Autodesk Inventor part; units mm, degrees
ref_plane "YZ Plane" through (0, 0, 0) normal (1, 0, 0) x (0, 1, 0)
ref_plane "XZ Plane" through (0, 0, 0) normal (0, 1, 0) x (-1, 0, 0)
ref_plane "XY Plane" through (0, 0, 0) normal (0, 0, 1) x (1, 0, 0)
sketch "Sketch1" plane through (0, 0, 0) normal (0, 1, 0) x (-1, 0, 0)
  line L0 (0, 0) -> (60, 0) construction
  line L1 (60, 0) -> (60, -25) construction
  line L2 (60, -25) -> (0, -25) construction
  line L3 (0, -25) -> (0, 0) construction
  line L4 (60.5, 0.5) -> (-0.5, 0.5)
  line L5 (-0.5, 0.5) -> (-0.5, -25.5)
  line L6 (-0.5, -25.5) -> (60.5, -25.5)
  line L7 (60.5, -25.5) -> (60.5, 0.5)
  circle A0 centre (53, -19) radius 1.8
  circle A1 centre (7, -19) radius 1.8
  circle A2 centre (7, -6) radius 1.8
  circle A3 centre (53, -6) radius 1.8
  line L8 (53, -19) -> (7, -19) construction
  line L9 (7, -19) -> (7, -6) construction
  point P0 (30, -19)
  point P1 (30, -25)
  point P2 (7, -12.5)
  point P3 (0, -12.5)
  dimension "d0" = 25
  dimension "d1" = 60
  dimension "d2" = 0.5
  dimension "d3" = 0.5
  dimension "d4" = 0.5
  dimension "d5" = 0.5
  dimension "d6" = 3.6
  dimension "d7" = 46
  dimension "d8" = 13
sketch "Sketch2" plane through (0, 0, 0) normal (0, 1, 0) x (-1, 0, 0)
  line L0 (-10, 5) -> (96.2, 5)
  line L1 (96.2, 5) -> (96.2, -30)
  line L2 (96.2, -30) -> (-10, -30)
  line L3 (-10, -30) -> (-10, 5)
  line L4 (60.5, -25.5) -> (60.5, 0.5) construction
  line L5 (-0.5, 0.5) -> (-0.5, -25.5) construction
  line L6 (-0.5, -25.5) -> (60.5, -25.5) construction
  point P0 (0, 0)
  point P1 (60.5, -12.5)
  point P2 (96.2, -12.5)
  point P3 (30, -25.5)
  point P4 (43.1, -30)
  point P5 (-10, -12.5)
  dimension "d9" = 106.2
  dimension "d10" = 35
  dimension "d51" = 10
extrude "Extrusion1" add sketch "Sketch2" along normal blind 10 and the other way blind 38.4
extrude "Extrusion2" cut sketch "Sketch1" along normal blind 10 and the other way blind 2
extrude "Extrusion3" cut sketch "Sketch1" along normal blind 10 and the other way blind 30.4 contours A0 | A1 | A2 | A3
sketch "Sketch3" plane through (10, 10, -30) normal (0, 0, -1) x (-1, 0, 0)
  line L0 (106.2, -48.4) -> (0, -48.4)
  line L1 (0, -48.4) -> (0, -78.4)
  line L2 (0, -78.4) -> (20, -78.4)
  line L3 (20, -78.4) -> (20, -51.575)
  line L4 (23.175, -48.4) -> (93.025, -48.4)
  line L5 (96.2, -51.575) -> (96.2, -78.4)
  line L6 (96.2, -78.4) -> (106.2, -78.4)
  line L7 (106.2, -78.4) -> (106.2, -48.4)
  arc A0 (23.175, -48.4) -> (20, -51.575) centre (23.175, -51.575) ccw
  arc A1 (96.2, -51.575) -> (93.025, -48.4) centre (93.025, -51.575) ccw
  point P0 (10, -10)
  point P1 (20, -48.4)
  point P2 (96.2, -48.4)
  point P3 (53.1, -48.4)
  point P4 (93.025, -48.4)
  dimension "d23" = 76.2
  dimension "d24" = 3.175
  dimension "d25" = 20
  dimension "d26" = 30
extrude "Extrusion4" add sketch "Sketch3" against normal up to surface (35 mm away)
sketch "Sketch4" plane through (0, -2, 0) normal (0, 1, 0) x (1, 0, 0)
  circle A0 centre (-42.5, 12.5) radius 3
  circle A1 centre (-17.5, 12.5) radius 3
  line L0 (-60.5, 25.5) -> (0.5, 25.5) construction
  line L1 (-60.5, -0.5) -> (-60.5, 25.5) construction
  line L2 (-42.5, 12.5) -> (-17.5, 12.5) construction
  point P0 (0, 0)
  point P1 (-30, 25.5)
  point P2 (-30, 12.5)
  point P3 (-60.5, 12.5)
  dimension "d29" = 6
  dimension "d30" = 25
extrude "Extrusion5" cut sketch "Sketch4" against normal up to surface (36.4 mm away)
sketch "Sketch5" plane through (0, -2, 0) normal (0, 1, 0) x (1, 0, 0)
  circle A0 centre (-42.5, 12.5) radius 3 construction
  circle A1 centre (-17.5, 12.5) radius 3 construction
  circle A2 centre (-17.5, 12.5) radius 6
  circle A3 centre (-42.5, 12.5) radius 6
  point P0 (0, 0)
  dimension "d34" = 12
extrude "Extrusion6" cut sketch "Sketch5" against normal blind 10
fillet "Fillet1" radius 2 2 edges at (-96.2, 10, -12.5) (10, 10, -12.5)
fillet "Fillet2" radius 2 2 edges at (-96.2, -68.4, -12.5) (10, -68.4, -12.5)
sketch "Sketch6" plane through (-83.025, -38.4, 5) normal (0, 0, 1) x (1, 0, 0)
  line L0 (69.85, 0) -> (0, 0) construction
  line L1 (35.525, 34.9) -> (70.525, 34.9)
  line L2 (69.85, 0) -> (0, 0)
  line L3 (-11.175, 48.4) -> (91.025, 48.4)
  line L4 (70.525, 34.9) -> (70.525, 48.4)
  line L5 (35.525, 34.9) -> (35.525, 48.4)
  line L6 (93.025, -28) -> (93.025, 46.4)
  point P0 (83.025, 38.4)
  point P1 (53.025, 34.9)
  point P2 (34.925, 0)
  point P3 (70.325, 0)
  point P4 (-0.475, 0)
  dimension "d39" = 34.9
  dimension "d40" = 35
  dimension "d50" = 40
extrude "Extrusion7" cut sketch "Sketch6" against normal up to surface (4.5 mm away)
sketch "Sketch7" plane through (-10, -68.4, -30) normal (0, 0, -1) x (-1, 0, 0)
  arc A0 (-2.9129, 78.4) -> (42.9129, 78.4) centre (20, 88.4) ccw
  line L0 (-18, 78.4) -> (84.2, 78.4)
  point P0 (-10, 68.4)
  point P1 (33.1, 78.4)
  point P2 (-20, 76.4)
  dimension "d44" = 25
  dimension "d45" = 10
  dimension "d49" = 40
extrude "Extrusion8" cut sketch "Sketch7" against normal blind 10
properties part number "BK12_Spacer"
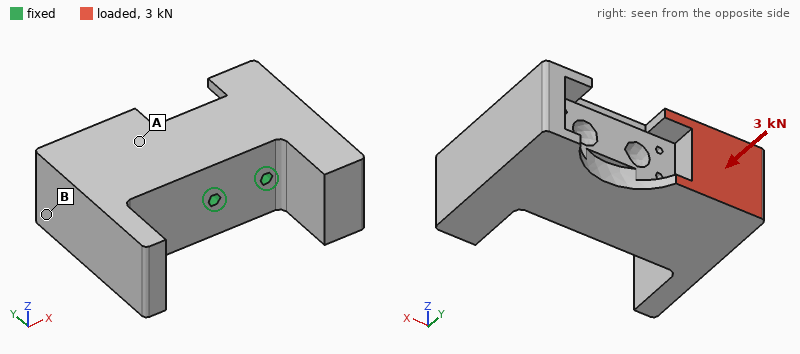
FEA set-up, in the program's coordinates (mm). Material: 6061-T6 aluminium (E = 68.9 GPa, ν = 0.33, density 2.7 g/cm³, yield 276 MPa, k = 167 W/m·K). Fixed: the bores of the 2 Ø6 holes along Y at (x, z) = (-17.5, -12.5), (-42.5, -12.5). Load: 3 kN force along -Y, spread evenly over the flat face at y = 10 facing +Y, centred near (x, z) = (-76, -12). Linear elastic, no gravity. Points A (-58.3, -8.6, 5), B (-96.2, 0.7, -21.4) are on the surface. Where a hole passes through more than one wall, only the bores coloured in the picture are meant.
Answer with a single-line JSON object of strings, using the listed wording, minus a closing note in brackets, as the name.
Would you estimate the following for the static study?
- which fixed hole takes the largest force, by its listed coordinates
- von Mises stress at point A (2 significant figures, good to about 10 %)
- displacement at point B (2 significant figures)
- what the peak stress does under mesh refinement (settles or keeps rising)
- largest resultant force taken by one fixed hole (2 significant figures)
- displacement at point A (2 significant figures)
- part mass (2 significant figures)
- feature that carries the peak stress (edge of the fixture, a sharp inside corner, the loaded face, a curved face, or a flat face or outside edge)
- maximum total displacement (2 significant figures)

{"which fixed hole takes the largest force, by its listed coordinates": "(-42.5, -12.5)", "von Mises stress at point A": "6.6 MPa", "displacement at point B": "22 µm", "what the peak stress does under mesh refinement": "keeps rising", "largest resultant force taken by one fixed hole": "4.2 kN", "displacement at point A": "7.3 µm", "part mass": "490 g", "feature that carries the peak stress": "edge of the fixture", "maximum total displacement": "25 µm"}
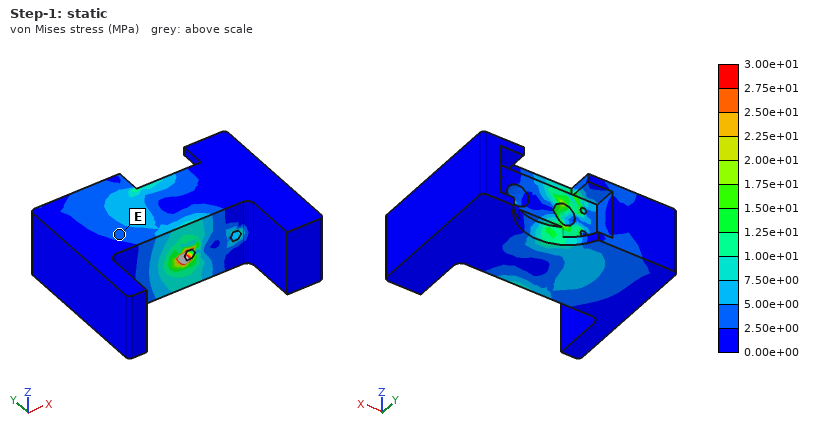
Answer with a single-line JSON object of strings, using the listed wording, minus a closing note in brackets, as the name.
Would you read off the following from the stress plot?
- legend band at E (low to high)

{"legend band at E": "2.50e+00 to 5.00e+00 MPa"}
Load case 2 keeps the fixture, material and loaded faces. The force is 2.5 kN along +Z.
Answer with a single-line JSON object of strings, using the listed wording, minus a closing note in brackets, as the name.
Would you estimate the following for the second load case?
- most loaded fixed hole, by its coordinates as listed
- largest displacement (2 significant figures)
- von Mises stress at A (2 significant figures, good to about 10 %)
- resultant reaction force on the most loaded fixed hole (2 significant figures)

{"most loaded fixed hole, by its coordinates as listed": "(-42.5, -12.5)", "largest displacement": "39 µm", "von Mises stress at A": "12 MPa", "resultant reaction force on the most loaded fixed hole": "5.0 kN"}
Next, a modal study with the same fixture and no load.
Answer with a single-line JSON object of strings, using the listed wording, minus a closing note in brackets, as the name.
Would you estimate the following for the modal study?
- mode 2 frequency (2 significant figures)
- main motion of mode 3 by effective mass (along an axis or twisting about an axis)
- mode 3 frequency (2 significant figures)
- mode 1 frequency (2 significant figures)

{"mode 2 frequency": "4100 Hz", "main motion of mode 3 by effective mass": "twisting about X", "mode 3 frequency": "5700 Hz", "mode 1 frequency": "4000 Hz"}
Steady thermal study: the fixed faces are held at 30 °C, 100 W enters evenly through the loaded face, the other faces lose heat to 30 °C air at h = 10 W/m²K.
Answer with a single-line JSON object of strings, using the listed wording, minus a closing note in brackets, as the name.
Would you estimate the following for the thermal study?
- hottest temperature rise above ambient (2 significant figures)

{"hottest temperature rise above ambient": "26 K"}
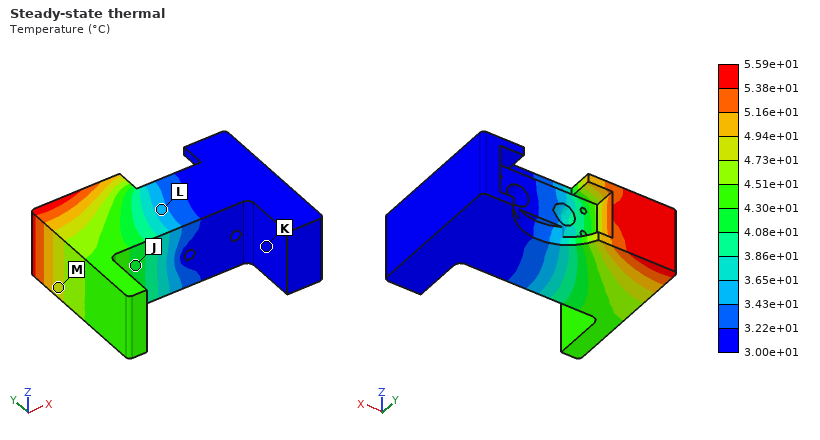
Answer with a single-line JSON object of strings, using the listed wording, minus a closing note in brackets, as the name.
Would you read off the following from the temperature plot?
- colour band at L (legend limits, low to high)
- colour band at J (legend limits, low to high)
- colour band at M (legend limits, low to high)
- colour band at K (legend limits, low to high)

{"colour band at L": "3.43e+01 to 3.65e+01 °C", "colour band at J": "4.08e+01 to 4.30e+01 °C", "colour band at M": "4.73e+01 to 4.94e+01 °C", "colour band at K": "3.00e+01 to 3.22e+01 °C"}
